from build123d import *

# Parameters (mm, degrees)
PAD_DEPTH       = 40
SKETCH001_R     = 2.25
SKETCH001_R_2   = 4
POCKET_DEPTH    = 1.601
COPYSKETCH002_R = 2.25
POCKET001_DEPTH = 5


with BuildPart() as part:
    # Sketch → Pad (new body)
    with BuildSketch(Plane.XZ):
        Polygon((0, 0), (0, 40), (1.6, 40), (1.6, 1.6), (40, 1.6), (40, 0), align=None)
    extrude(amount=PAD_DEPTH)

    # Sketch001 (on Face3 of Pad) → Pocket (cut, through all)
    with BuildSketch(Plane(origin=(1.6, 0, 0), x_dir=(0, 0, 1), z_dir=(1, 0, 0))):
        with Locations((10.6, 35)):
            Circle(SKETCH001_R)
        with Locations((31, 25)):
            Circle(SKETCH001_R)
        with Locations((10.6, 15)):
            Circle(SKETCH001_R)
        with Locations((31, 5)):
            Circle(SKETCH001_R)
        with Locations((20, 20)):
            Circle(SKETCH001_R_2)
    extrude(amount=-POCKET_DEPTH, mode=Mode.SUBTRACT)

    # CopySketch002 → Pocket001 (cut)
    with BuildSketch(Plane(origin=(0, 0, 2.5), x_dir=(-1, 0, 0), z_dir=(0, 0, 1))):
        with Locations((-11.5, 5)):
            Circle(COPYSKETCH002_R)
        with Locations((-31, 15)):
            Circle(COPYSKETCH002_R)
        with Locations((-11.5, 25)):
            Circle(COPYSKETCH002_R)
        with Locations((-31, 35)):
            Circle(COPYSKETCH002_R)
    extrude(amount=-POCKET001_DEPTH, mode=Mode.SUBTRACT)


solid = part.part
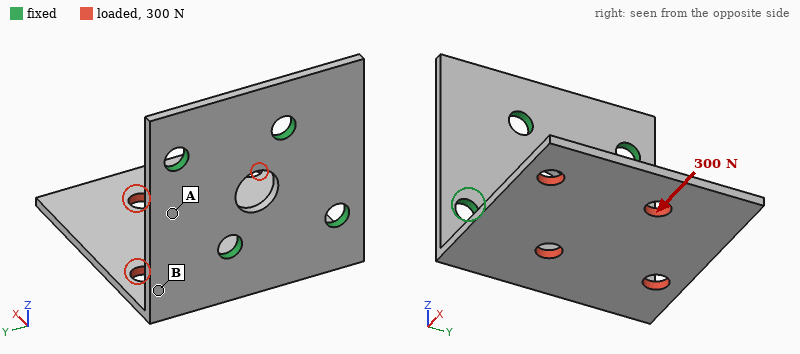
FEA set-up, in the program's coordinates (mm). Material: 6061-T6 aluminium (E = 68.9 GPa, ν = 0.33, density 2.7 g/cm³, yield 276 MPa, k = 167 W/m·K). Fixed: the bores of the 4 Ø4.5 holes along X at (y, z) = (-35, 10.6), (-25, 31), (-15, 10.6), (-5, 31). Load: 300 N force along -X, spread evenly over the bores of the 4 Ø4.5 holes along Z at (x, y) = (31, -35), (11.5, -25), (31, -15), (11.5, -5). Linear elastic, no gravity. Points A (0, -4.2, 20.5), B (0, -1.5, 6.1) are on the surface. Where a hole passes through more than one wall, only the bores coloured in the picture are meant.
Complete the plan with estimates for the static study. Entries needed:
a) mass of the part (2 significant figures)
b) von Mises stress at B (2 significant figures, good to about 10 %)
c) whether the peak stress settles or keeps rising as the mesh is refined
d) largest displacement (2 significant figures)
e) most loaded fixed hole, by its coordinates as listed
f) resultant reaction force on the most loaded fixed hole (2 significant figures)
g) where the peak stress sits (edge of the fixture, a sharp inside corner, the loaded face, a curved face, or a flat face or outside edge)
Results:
13 g
46 MPa
keeps rising
0.52 mm
(-15, 10.6)
230 N
edge of the fixture
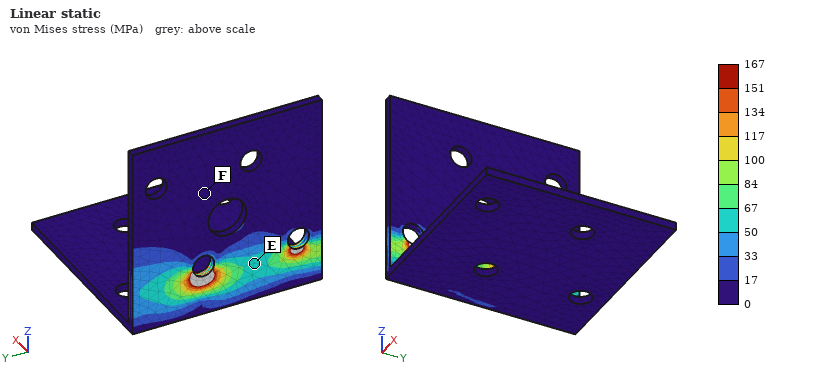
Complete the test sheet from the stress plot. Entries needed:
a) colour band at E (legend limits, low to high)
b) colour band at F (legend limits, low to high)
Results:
50 to 67 MPa
0 to 17 MPa
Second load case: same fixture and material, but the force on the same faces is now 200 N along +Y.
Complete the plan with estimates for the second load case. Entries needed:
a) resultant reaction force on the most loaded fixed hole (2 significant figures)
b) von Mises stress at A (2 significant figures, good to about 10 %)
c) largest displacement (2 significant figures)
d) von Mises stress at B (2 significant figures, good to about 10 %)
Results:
220 N
18 MPa
0.30 mm
25 MPa
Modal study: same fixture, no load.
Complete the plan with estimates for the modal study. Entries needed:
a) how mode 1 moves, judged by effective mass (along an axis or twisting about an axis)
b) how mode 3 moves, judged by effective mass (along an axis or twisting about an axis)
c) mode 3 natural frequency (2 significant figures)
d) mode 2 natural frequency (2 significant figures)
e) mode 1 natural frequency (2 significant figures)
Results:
along Z
along Y
2400 Hz
1700 Hz
640 Hz
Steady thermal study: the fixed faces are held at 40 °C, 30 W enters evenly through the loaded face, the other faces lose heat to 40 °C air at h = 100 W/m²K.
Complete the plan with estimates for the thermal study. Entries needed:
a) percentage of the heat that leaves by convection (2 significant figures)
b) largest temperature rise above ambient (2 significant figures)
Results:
45 %
58 K
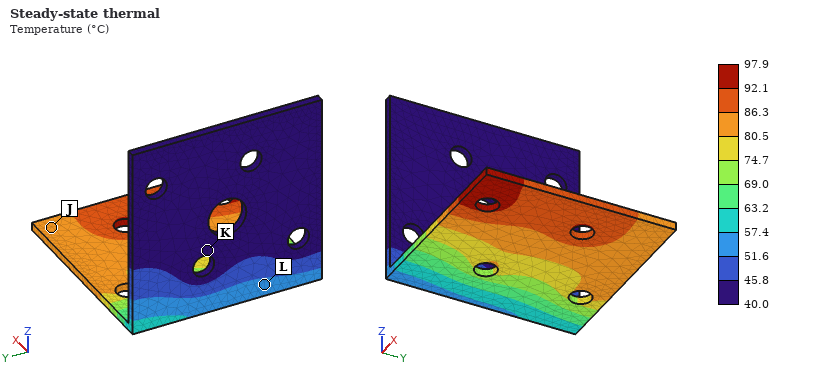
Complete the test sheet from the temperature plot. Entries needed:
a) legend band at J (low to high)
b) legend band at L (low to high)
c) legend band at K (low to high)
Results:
80.5 to 86.3 °C
51.6 to 57.4 °C
40.0 to 45.8 °C
